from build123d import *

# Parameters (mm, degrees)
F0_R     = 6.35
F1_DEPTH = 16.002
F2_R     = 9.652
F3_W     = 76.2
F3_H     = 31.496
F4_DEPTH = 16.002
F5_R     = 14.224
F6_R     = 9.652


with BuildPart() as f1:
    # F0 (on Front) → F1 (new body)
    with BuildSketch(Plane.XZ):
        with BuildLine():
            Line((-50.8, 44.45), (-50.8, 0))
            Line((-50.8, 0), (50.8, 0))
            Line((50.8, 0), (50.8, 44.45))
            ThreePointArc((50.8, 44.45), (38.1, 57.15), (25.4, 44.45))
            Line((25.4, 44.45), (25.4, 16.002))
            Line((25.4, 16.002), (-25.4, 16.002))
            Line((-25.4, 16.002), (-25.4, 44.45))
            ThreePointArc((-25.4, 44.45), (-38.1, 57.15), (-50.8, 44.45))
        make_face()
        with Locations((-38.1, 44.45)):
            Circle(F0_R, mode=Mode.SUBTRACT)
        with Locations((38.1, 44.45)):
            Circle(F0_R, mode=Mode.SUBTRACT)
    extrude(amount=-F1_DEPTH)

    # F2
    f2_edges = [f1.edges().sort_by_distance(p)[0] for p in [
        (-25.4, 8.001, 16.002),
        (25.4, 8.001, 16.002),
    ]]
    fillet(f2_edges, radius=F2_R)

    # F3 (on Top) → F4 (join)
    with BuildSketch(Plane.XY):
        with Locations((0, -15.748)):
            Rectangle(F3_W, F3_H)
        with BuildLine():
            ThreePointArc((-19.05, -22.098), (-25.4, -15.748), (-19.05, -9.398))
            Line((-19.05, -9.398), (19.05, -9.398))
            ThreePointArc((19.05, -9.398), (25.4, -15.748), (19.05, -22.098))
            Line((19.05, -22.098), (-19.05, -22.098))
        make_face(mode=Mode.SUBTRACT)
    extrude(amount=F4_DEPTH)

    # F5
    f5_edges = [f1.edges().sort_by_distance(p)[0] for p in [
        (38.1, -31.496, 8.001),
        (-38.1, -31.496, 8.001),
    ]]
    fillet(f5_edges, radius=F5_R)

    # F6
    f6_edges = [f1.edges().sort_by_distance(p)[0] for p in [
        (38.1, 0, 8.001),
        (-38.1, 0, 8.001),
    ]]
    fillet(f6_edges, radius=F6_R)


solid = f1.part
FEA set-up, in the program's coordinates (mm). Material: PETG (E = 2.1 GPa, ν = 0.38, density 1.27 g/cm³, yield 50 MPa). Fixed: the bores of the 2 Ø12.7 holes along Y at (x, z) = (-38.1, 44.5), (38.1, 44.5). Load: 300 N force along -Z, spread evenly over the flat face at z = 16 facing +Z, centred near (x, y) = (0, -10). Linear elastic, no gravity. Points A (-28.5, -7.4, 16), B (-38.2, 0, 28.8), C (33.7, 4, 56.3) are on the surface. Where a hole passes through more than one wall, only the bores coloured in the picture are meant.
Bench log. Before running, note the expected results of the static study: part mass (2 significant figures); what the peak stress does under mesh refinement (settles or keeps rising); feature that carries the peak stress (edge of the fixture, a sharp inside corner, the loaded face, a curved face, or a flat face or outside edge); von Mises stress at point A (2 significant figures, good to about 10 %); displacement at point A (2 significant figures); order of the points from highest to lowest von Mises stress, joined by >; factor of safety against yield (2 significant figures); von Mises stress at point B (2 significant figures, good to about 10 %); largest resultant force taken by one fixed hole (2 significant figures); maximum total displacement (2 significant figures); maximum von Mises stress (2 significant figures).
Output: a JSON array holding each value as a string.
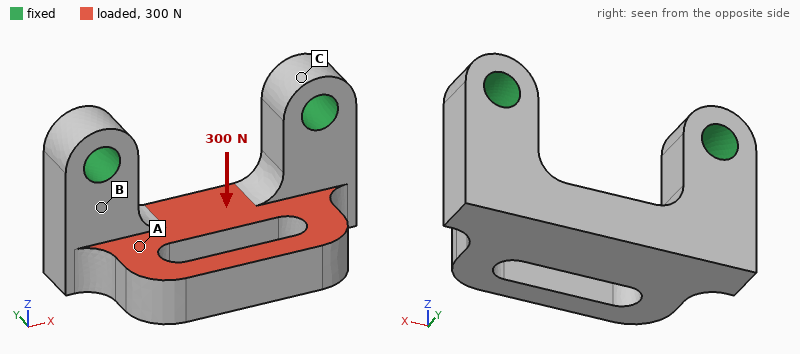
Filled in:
["100 g", "settles", "a curved face", "1.5 MPa", "0.091 mm", "B > A > C", "10", "2.9 MPa", "160 N", "0.29 mm", "4.8 MPa"]
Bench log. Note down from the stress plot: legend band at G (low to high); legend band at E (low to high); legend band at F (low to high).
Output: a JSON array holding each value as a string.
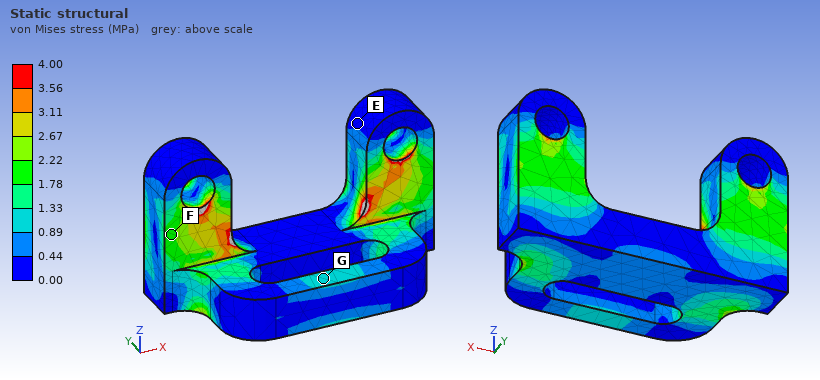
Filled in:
["0.89 to 1.33 MPa", "0.00 to 0.44 MPa", "1.78 to 2.22 MPa"]
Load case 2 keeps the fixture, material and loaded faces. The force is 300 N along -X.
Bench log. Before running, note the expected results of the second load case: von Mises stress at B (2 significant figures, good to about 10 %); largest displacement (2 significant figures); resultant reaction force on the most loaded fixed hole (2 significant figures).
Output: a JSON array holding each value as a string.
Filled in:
["1.6 MPa", "0.11 mm", "160 N"]
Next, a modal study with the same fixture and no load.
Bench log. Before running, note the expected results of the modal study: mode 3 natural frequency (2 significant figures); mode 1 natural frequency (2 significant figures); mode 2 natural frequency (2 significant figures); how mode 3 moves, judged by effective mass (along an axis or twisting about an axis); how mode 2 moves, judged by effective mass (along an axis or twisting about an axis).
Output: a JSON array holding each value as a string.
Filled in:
["1700 Hz", "730 Hz", "1300 Hz", "along Y", "along X"]
